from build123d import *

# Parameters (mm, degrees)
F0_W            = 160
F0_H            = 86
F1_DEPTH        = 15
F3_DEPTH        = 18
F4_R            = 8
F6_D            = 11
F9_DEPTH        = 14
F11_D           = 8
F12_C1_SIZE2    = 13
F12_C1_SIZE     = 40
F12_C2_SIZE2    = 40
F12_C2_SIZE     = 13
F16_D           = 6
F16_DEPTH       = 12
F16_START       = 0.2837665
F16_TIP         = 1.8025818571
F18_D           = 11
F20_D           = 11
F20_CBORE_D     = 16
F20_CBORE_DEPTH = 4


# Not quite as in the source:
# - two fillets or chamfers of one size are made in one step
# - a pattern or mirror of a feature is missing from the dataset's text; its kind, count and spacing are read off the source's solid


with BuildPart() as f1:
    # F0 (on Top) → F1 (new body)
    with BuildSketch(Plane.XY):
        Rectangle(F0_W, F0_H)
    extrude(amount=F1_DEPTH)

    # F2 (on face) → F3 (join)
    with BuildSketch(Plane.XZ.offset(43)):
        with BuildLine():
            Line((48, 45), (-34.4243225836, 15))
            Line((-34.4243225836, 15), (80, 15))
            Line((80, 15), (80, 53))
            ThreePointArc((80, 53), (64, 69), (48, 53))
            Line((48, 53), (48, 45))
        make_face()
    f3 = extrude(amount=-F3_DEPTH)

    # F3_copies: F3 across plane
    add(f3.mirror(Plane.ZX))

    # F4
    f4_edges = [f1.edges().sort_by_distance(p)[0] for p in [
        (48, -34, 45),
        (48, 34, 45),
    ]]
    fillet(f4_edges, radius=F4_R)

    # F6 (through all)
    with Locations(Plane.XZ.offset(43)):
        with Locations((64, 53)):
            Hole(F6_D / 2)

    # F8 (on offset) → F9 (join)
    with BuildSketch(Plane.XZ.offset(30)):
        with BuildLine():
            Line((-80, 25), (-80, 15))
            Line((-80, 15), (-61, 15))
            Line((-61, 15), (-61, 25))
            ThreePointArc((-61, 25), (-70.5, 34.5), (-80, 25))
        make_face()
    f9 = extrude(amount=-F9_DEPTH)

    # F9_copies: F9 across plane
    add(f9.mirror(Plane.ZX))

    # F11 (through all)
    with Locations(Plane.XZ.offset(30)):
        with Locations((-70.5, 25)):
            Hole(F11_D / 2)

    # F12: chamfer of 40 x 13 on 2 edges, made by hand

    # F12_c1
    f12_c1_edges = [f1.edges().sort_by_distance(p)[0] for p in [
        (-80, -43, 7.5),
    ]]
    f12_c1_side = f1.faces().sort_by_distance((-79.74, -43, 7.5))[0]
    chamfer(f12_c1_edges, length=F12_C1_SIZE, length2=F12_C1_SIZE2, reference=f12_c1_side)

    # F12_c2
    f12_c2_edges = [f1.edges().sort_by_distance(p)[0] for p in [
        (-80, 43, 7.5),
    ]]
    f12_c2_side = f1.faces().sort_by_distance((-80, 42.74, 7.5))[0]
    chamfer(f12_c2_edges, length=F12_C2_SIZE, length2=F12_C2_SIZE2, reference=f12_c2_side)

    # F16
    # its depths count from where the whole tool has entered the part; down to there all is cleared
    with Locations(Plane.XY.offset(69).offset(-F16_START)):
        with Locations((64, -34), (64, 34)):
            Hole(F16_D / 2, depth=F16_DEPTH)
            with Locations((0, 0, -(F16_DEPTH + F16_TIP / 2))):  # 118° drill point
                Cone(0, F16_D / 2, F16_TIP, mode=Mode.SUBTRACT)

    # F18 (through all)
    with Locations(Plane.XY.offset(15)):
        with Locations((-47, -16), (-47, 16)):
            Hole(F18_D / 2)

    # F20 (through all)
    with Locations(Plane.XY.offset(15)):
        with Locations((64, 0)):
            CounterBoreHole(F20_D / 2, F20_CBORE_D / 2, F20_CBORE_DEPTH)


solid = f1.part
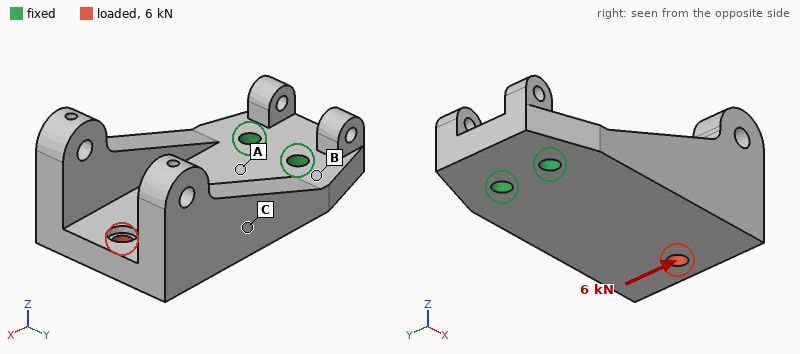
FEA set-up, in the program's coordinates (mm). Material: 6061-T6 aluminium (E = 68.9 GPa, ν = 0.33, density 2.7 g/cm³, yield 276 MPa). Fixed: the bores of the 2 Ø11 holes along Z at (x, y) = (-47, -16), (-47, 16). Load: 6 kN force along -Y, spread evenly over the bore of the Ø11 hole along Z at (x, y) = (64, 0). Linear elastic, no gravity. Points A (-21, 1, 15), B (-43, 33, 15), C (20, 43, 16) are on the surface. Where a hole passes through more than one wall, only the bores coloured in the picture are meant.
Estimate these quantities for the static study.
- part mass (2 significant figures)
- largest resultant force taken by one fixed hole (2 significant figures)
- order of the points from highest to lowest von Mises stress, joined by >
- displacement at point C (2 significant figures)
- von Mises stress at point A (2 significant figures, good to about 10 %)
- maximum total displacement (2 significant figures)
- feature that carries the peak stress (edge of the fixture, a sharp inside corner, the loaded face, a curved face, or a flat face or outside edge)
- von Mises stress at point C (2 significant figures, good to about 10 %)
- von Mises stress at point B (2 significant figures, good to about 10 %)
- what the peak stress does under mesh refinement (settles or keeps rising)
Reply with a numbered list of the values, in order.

1. 810 g
2. 17 kN
3. B > A > C
4. 0.069 mm
5. 16 MPa
6. 0.13 mm
7. edge of the fixture
8. 7.8 MPa
9. 26 MPa
10. keeps rising
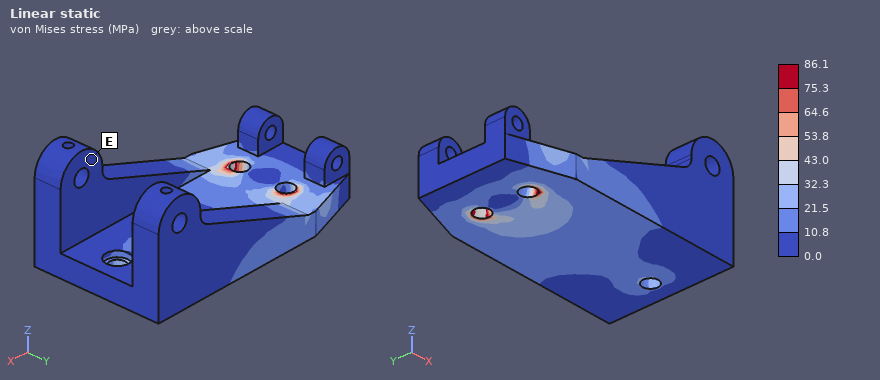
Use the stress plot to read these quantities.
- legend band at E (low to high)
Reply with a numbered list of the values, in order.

1. 0.0 to 10.8 MPa
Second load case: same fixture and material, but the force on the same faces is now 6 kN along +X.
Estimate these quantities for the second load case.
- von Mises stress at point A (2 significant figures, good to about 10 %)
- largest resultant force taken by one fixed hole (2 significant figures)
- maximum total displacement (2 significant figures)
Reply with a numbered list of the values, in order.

1. 2.6 MPa
2. 3.0 kN
3. 47 µm
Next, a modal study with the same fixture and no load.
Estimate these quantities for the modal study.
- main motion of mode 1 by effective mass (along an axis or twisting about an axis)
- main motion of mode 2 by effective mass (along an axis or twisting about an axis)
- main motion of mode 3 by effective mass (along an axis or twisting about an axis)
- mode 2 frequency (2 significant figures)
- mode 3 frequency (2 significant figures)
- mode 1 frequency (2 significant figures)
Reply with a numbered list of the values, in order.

1. along Z
2. along Y
3. along Y
4. 1300 Hz
5. 2000 Hz
6. 600 Hz
